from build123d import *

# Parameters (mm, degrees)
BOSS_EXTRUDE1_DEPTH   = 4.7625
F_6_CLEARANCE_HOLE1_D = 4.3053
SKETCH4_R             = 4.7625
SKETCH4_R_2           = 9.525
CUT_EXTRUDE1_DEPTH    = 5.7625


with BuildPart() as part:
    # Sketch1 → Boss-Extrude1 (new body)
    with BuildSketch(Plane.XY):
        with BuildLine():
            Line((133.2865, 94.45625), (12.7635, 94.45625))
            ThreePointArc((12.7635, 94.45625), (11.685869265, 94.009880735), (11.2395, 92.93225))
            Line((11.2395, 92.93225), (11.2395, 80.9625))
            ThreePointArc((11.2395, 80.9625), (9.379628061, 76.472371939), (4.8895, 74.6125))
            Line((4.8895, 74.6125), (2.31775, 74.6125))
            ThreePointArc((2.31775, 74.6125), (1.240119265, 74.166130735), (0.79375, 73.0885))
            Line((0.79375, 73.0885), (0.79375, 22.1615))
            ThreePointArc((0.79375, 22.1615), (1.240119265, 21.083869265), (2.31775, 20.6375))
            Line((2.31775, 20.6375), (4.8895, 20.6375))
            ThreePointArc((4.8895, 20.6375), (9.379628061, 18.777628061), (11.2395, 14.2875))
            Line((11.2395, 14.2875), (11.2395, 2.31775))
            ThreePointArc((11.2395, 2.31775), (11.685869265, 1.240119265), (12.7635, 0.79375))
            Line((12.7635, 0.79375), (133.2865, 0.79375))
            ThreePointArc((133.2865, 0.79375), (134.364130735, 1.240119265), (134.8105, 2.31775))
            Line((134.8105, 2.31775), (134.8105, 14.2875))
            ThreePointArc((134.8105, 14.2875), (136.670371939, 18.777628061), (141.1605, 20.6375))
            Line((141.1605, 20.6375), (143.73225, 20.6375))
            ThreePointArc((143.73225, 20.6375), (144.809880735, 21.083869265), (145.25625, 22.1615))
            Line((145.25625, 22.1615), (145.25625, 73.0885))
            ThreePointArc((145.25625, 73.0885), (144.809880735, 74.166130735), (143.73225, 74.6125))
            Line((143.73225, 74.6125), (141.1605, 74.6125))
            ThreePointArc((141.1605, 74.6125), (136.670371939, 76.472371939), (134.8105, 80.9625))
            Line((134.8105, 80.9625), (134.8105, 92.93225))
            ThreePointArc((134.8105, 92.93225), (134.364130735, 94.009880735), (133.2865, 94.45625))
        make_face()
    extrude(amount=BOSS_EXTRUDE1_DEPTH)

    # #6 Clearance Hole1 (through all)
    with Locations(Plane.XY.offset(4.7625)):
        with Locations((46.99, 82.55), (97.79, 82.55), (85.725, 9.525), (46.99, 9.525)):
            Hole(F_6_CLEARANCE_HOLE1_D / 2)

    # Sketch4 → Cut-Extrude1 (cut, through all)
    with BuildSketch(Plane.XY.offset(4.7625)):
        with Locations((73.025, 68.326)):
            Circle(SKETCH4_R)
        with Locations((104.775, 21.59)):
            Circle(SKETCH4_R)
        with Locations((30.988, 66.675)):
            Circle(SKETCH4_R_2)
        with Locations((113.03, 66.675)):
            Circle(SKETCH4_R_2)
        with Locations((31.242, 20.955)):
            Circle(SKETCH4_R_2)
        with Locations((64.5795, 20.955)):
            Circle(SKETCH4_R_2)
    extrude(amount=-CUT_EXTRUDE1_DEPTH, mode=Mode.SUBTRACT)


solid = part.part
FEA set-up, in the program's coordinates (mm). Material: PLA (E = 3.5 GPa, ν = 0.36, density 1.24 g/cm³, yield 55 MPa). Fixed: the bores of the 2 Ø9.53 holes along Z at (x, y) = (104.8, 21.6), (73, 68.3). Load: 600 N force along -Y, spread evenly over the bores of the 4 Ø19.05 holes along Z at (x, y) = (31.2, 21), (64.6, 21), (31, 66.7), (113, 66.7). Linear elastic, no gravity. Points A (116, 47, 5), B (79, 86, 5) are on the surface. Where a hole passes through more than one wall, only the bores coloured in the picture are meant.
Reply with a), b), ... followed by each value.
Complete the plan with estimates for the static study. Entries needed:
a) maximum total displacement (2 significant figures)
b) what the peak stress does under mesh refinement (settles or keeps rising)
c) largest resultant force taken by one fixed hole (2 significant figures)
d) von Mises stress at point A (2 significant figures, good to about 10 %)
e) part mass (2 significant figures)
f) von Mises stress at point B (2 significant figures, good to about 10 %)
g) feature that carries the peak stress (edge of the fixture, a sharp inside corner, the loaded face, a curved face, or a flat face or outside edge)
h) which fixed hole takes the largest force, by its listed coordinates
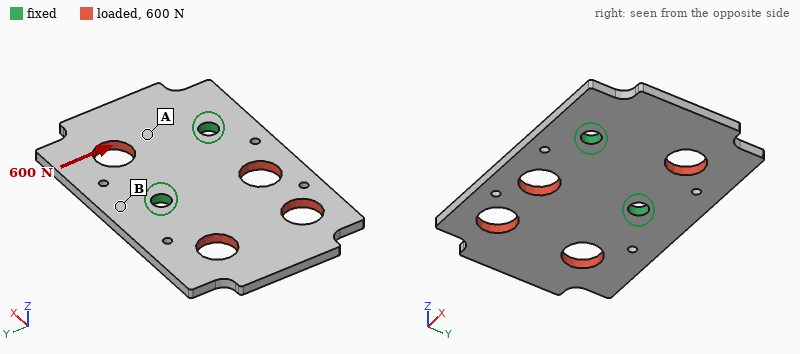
a) 0.11 mm
b) keeps rising
c) 520 N
d) 0.58 MPa
e) 67 g
f) 1.6 MPa
g) edge of the fixture
h) (73, 68.3)
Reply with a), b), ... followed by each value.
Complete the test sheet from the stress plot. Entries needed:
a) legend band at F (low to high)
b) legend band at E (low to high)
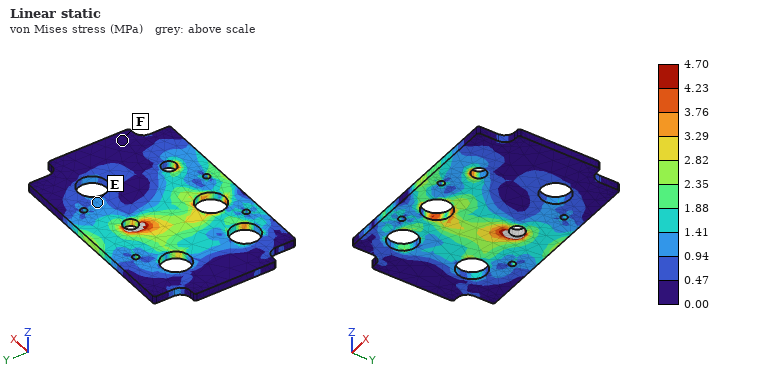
a) 0.00 to 0.47 MPa
b) 0.94 to 1.41 MPa
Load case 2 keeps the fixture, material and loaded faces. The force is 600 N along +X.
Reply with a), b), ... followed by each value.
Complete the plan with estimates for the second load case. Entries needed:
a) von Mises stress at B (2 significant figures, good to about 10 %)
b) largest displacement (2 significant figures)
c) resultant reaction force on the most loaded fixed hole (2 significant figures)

a) 0.32 MPa
b) 47 µm
c) 300 N
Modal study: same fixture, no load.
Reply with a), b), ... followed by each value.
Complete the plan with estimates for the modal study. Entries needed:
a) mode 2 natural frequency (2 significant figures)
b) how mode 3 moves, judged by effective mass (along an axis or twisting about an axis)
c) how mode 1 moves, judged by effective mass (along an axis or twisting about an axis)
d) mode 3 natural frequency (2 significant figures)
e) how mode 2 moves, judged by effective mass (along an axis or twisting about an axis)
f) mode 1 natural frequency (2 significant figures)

a) 450 Hz
b) along Z
c) along Z
d) 470 Hz
e) twisting about X
f) 230 Hz
